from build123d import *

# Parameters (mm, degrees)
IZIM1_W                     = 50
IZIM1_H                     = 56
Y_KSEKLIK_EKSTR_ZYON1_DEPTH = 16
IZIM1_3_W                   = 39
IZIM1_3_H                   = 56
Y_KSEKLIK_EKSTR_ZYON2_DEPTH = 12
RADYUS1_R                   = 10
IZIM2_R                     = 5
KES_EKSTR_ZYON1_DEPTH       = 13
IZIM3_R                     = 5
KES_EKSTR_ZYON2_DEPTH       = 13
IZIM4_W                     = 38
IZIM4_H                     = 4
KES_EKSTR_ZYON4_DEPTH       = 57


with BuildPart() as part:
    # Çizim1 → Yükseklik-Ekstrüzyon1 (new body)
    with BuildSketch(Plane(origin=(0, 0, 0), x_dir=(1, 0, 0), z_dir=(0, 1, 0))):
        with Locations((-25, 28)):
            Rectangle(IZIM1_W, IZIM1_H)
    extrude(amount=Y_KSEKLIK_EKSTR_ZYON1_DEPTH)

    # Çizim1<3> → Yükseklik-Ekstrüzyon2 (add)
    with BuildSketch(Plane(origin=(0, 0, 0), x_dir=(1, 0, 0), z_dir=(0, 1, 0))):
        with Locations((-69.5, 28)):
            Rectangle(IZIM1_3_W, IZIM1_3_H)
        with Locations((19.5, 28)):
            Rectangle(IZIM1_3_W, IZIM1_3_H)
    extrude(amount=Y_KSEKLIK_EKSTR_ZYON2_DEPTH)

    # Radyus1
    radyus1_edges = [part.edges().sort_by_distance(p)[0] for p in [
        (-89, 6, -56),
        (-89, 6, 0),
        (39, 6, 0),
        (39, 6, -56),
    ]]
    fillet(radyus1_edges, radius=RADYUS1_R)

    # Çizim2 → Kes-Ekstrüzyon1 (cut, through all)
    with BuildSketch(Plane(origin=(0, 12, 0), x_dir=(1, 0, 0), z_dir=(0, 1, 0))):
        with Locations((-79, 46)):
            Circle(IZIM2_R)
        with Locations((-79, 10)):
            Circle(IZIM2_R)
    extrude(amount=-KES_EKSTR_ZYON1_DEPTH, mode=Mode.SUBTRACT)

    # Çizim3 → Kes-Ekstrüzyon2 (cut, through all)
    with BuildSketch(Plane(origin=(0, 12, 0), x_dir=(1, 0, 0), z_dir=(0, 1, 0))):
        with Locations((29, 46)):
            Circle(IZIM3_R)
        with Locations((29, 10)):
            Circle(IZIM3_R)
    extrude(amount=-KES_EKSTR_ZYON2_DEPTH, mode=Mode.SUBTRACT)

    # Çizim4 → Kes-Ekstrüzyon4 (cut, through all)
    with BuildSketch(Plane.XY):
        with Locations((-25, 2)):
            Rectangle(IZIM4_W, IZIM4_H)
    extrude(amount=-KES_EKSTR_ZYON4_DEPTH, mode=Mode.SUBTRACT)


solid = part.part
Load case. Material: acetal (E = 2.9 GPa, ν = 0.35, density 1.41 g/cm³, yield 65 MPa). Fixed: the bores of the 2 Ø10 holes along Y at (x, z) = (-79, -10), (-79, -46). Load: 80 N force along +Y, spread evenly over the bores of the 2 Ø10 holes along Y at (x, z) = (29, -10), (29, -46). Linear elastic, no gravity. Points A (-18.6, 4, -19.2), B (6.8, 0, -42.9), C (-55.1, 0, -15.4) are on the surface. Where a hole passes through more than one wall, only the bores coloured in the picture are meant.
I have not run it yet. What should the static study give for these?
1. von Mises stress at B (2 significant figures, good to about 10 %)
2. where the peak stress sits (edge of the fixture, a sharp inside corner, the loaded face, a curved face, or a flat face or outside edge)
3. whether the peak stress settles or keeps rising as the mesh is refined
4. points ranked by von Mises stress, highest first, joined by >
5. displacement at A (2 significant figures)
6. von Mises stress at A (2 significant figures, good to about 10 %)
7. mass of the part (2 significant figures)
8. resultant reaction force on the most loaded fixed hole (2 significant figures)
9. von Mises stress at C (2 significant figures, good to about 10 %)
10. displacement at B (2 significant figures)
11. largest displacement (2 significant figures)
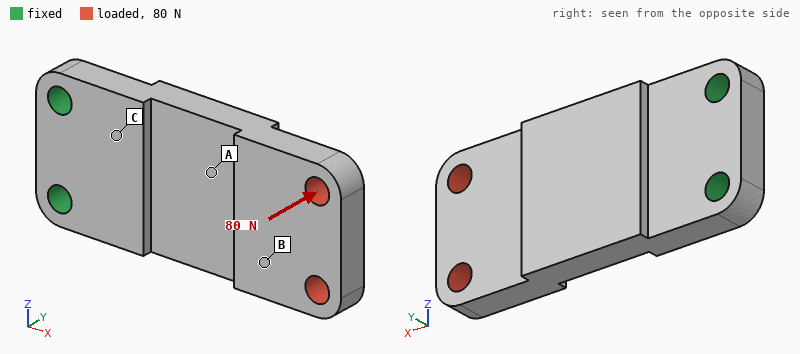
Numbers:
1.3 MPa
edge of the fixture
keeps rising
C > A > B
0.53 mm
2.8 MPa
120 g
41 N
4.6 MPa
0.98 mm
1.6 mm
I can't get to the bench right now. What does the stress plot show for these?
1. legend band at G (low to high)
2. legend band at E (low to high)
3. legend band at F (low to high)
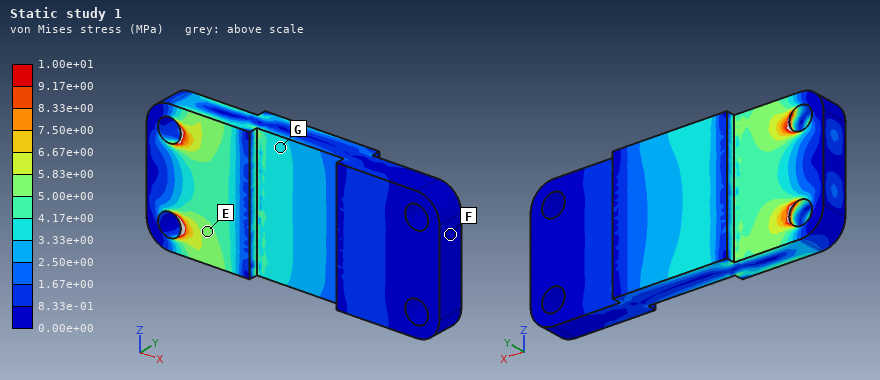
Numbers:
3.33e+00 to 4.17e+00 MPa
5.00e+00 to 5.83e+00 MPa
0.00e+00 to 8.33e-01 MPa
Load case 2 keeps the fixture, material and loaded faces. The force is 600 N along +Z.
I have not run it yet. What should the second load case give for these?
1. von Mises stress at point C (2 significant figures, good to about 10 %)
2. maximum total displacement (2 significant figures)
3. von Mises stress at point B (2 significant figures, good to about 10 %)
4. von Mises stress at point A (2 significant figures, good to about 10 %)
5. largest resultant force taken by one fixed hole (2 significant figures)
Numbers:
5.0 MPa
0.80 mm
1.4 MPa
4.0 MPa
1.6 kN
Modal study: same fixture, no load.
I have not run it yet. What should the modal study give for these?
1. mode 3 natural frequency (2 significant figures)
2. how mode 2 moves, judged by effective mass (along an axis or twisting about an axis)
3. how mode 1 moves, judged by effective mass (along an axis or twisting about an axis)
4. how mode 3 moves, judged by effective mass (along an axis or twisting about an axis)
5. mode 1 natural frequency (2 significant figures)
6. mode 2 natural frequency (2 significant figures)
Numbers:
940 Hz
along Z
along Y
along Z
210 Hz
760 Hz
